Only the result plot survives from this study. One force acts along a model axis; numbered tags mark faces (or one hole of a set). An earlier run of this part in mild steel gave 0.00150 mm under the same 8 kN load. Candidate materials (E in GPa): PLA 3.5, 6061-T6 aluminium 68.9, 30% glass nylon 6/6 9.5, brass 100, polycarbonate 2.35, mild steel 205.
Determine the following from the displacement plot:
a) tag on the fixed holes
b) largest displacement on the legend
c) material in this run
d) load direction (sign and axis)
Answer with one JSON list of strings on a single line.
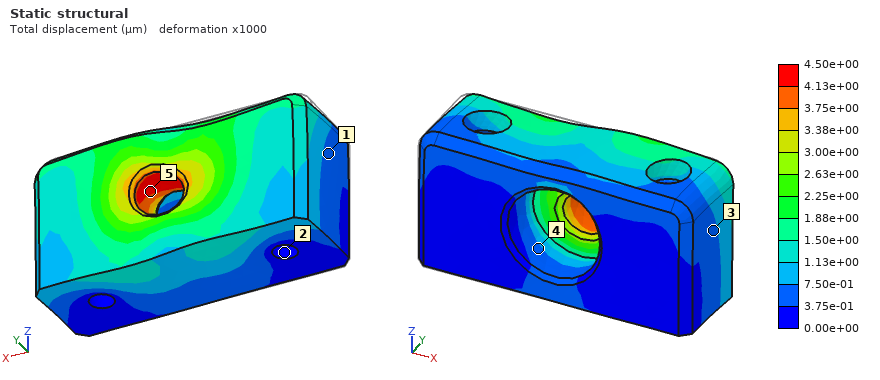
["2", "4.50e+00 µm", "6061-T6 aluminium", "+X"]
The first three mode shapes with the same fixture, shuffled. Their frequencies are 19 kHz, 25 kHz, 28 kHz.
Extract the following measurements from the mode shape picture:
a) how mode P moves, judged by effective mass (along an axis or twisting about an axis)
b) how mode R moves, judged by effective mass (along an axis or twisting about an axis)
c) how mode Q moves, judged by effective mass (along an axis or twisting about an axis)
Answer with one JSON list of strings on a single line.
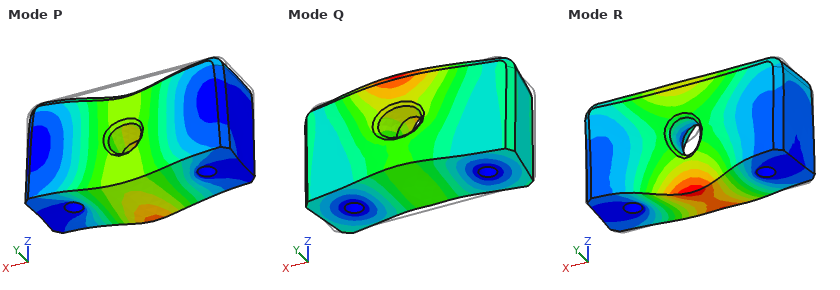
["along Z", "twisting about X", "along Y"]
